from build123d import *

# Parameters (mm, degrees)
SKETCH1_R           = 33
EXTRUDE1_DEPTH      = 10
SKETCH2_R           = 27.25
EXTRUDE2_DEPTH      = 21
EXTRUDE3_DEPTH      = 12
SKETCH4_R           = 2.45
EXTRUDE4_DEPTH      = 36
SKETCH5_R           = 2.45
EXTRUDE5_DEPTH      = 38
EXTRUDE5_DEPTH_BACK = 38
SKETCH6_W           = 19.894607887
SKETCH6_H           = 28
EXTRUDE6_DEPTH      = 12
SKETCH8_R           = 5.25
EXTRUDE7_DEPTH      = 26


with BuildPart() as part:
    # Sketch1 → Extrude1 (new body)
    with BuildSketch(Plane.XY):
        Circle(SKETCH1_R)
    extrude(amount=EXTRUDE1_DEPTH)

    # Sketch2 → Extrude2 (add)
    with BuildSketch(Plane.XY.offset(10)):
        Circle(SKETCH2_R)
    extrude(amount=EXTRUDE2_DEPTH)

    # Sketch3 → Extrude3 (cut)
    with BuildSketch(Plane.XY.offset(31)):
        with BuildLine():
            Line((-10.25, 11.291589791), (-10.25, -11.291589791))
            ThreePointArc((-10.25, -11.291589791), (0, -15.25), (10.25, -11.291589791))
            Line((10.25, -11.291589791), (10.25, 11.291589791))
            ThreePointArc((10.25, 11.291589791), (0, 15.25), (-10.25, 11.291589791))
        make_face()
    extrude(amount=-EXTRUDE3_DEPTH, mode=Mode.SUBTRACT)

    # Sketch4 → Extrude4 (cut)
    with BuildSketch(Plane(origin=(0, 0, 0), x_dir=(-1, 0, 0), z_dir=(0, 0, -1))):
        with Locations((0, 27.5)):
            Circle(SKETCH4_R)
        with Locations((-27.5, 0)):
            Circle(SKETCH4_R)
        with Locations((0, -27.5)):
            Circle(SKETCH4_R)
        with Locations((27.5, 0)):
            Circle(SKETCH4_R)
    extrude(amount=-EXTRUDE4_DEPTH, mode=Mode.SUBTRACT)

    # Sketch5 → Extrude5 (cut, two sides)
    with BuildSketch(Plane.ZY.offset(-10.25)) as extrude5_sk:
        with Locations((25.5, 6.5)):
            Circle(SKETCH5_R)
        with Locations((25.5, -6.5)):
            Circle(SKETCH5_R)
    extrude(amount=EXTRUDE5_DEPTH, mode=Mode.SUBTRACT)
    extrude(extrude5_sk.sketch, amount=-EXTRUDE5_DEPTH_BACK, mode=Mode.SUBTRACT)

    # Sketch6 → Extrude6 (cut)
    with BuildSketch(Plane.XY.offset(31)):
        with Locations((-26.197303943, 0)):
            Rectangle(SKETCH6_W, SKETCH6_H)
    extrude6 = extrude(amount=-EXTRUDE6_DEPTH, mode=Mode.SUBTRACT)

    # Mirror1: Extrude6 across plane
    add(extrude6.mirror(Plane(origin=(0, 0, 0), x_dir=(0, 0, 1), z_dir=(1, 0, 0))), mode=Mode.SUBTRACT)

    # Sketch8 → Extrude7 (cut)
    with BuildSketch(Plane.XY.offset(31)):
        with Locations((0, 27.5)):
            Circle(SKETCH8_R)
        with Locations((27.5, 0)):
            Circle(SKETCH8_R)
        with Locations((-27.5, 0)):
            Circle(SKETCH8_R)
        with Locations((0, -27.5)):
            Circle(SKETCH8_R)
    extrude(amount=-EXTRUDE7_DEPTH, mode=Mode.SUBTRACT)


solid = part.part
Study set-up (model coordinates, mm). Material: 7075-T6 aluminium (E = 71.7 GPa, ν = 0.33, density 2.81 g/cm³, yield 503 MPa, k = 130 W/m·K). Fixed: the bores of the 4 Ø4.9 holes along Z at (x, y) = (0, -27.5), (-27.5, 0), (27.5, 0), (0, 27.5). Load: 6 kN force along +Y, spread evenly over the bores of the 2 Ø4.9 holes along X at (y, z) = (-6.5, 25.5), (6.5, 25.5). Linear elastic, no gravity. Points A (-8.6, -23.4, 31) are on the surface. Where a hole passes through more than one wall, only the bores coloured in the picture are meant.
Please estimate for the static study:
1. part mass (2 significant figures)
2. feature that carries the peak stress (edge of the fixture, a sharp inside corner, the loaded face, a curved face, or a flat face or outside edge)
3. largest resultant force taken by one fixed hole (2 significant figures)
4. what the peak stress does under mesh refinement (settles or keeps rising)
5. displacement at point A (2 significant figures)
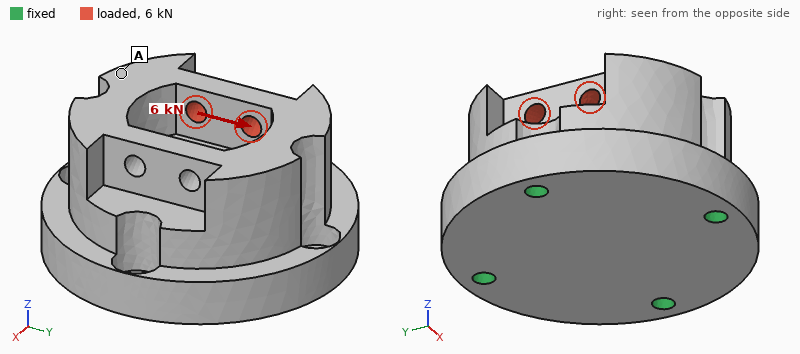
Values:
180 g
edge of the fixture
3.3 kN
keeps rising
22 µm
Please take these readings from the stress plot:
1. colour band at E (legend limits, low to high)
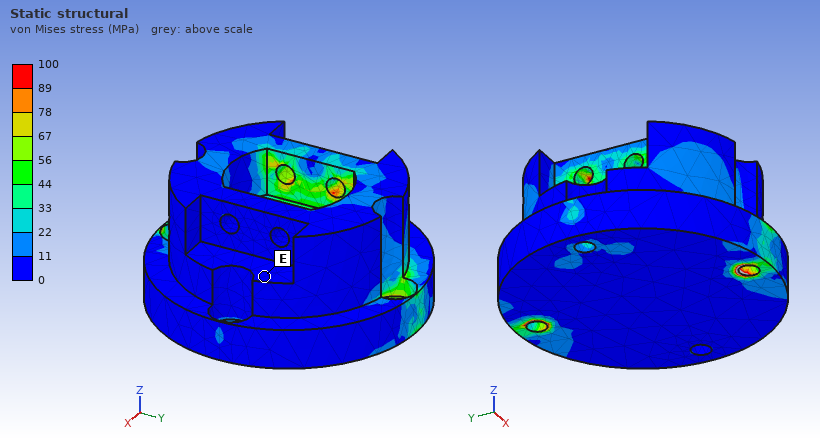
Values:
0 to 11 MPa
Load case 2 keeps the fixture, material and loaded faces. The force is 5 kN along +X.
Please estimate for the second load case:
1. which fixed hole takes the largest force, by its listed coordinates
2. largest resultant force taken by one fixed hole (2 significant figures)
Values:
(-27.5, 0)
2.9 kN
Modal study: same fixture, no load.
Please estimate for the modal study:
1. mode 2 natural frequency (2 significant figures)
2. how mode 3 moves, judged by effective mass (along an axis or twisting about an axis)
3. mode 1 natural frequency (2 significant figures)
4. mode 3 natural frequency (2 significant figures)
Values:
12 kHz
along Z
12 kHz
13 kHz
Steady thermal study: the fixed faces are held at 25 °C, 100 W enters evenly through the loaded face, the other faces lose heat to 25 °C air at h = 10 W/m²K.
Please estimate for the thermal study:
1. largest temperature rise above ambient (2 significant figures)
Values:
58 K
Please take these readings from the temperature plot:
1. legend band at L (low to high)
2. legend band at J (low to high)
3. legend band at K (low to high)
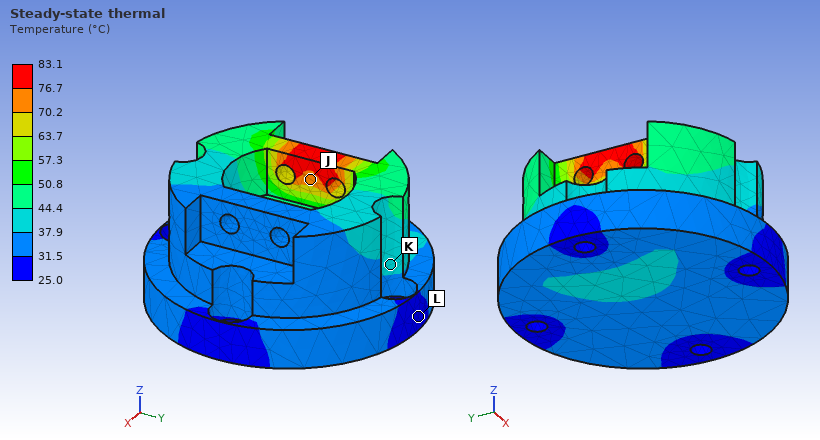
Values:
25.0 to 31.5 °C
70.2 to 76.7 °C
37.9 to 44.4 °C
